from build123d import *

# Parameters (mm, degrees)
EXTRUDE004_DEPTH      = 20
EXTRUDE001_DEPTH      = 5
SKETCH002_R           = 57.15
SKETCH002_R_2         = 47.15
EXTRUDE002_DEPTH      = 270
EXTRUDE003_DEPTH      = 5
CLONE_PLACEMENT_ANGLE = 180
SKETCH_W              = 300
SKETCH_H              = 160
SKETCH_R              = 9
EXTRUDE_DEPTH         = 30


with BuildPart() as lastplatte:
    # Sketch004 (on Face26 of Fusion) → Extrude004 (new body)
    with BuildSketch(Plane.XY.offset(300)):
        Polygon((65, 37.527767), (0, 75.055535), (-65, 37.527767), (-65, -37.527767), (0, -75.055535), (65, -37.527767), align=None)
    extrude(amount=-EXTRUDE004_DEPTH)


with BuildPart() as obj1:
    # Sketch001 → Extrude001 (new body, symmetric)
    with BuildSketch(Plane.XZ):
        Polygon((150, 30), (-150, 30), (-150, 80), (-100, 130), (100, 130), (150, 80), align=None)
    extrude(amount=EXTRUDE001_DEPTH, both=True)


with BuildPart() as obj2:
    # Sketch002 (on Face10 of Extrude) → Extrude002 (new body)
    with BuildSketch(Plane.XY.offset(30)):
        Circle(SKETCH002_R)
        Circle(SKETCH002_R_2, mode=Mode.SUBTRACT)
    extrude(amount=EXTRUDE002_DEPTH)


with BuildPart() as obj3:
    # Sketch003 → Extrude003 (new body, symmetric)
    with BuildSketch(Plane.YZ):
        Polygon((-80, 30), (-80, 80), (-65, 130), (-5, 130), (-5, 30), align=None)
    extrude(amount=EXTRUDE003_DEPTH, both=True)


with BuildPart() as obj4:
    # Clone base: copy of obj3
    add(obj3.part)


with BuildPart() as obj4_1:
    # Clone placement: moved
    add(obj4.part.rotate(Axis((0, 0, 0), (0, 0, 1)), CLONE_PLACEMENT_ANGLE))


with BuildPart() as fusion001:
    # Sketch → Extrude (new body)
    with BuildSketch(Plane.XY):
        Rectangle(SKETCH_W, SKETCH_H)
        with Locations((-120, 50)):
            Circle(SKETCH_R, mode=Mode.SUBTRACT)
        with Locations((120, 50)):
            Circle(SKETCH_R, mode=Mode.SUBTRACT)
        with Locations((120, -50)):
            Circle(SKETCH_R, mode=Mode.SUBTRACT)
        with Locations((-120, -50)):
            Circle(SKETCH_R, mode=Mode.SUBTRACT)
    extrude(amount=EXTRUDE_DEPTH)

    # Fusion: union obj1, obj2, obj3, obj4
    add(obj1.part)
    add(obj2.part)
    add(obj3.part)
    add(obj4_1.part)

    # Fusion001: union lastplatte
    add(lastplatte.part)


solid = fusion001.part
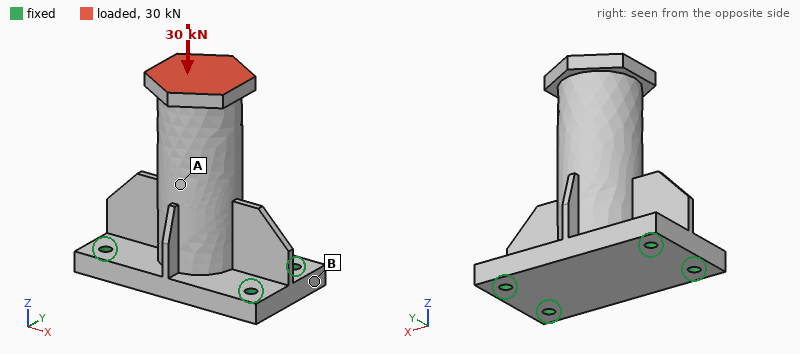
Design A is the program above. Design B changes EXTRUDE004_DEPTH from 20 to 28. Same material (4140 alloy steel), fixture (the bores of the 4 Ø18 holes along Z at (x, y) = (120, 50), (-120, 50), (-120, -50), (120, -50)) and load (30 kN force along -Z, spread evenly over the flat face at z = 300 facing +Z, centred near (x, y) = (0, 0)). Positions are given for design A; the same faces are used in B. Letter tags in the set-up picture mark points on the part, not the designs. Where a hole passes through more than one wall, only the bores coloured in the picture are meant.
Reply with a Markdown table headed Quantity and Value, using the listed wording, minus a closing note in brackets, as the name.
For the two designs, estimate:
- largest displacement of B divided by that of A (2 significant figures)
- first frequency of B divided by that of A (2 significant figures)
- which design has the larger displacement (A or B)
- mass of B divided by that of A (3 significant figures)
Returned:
| Quantity | Value |
|---|---|
| largest displacement of B divided by that of A | 0.91 |
| first frequency of B divided by that of A | 0.93 |
| which design has the larger displacement | A |
| mass of B divided by that of A | 1.03 |
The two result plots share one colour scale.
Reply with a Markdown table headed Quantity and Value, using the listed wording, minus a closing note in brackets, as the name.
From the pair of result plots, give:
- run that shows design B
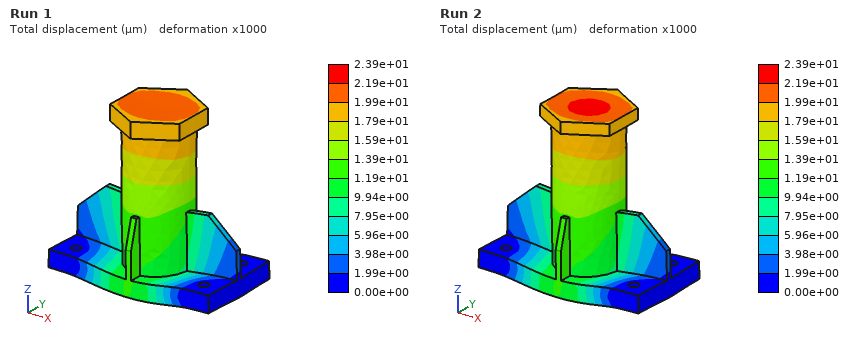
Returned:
| Quantity | Value |
|---|---|
| run that shows design B | Run 1 |
